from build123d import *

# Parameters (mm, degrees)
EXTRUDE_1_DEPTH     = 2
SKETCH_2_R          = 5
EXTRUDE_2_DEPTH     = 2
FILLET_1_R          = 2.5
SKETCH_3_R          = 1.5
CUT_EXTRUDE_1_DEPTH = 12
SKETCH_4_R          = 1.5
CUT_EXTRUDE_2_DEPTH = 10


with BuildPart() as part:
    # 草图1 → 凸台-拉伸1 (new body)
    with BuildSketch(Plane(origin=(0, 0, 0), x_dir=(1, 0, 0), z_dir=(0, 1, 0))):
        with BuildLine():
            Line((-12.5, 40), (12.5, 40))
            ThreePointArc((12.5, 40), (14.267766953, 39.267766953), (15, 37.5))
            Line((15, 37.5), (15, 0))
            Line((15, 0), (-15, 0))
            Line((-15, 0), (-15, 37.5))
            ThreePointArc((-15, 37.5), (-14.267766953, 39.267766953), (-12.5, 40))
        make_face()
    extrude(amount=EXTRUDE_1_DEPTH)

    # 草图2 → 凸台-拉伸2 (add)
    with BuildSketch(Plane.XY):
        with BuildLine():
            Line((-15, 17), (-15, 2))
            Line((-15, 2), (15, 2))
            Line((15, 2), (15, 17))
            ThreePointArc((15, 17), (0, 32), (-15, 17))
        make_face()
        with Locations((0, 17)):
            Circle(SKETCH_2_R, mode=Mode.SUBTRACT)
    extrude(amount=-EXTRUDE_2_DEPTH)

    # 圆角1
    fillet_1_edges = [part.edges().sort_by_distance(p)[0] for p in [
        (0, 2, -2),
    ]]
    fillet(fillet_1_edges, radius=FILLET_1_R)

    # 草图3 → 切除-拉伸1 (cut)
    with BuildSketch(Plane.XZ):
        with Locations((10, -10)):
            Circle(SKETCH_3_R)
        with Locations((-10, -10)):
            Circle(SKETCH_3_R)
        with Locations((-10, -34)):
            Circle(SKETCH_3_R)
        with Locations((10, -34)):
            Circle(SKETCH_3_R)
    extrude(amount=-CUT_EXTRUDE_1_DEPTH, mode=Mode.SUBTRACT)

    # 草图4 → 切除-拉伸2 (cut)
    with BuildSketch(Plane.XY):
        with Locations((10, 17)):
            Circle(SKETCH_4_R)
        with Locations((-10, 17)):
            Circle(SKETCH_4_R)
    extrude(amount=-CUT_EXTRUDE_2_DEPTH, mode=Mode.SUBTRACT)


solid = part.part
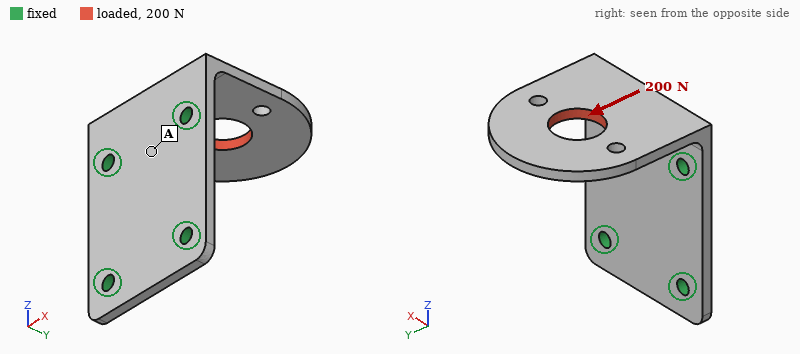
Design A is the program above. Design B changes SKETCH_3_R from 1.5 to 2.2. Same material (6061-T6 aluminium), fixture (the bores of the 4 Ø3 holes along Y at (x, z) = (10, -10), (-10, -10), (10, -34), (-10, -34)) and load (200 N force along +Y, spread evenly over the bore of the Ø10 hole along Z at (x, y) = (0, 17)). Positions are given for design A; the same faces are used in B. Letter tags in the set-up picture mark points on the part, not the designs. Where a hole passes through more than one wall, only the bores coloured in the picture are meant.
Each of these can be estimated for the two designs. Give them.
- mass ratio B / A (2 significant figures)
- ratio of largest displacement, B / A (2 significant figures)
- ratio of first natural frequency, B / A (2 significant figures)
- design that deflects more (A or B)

0.98
0.80
1.0
A
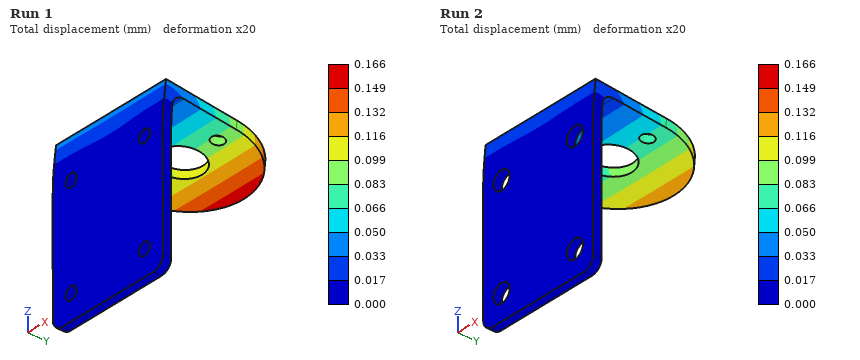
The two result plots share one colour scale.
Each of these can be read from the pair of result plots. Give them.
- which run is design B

Run 2
